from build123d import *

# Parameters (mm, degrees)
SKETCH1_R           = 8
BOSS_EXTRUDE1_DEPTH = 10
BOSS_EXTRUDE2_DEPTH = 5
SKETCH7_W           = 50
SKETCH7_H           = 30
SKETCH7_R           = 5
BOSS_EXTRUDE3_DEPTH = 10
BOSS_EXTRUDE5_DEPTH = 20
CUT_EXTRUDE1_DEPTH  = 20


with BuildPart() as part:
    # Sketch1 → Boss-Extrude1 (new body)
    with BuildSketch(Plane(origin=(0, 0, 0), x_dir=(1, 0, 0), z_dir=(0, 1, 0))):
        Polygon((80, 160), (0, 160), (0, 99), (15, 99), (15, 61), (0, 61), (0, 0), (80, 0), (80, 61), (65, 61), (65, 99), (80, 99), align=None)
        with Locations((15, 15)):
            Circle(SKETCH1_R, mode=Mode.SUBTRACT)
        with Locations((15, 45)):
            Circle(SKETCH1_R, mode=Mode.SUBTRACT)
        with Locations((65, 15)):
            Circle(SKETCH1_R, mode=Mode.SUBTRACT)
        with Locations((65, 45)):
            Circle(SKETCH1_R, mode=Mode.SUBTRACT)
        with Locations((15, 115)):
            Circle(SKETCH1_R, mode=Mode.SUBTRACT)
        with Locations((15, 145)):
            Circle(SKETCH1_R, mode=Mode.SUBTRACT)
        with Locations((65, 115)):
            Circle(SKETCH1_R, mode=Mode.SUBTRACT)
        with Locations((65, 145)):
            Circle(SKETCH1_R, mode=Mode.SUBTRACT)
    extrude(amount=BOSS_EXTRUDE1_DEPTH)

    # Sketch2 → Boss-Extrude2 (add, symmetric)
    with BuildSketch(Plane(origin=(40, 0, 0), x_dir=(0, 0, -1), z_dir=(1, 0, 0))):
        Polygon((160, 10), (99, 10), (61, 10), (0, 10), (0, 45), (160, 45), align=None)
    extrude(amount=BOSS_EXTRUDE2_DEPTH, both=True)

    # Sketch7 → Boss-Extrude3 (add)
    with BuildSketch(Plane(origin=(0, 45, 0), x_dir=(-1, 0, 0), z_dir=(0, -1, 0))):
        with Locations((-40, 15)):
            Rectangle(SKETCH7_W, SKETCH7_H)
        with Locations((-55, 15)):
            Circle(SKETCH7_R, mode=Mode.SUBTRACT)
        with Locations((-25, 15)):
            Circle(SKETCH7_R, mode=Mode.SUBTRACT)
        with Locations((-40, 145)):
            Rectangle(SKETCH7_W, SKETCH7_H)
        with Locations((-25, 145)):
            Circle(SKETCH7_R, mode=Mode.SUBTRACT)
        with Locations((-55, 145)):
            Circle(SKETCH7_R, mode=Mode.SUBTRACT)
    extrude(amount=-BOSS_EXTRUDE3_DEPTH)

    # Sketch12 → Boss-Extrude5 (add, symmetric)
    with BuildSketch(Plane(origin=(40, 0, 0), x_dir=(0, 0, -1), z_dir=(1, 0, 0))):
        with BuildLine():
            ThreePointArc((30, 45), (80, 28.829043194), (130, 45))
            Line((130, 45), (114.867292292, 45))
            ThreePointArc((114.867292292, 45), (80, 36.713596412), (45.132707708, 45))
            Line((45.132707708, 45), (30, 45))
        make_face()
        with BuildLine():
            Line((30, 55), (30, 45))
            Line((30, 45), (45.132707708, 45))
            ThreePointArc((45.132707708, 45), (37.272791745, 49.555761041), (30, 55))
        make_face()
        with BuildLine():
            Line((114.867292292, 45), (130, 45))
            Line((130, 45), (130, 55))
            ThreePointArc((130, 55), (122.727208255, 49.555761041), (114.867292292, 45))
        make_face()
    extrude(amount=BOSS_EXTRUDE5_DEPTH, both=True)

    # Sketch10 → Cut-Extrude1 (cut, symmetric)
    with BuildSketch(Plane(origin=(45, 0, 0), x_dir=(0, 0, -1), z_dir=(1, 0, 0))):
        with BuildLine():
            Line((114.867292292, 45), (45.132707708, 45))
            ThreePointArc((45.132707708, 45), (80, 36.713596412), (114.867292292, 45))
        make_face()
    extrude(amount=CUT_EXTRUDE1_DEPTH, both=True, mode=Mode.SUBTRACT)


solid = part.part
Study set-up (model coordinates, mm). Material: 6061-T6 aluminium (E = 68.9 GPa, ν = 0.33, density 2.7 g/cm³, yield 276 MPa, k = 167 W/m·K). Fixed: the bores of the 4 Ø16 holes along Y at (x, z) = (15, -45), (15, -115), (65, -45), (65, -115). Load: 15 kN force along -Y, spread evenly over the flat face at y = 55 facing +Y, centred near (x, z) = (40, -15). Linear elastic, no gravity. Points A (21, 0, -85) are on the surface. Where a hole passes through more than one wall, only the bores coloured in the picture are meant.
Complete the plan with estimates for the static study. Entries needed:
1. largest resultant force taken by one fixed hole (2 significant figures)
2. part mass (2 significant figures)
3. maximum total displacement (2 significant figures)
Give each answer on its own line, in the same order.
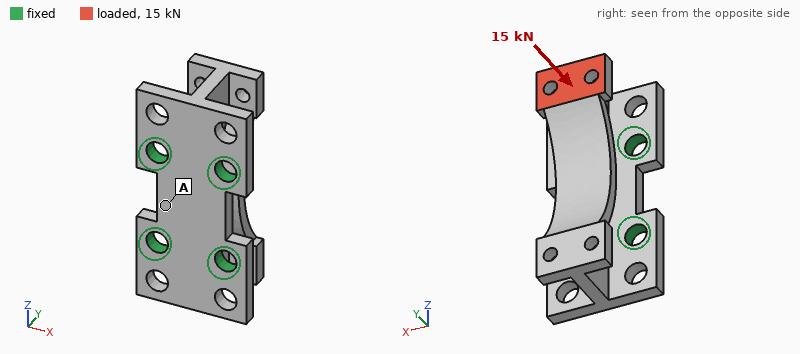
10 kN
560 g
0.25 mm
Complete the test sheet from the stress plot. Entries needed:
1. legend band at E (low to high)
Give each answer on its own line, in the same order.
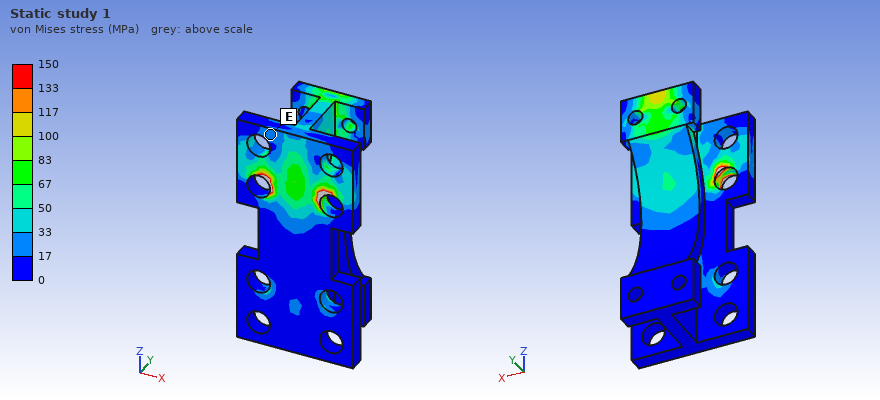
17 to 33 MPa
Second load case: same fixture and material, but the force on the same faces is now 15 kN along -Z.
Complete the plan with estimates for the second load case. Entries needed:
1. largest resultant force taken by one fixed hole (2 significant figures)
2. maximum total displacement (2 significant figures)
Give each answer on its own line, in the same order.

6.9 kN
0.22 mm
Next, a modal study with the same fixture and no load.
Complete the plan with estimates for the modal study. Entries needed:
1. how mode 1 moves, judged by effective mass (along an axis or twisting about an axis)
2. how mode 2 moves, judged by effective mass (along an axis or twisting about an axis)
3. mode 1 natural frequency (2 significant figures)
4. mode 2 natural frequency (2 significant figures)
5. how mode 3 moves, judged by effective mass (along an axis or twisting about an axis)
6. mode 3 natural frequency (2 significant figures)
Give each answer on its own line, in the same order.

along X
twisting about Y
2200 Hz
2300 Hz
along Z
4100 Hz
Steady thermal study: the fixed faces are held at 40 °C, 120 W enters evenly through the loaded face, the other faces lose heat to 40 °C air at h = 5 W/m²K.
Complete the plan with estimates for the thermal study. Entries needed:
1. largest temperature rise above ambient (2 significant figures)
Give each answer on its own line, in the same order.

69 K
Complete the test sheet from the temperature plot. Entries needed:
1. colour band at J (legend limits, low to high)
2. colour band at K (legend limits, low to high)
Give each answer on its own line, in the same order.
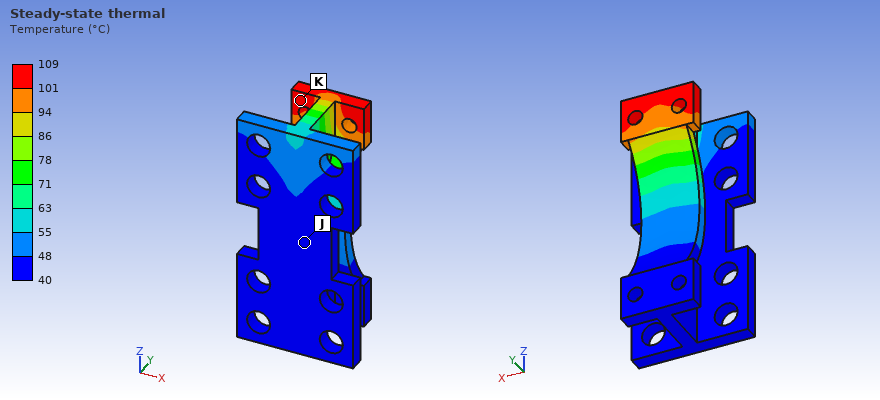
40 to 48 °C
101 to 109 °C
